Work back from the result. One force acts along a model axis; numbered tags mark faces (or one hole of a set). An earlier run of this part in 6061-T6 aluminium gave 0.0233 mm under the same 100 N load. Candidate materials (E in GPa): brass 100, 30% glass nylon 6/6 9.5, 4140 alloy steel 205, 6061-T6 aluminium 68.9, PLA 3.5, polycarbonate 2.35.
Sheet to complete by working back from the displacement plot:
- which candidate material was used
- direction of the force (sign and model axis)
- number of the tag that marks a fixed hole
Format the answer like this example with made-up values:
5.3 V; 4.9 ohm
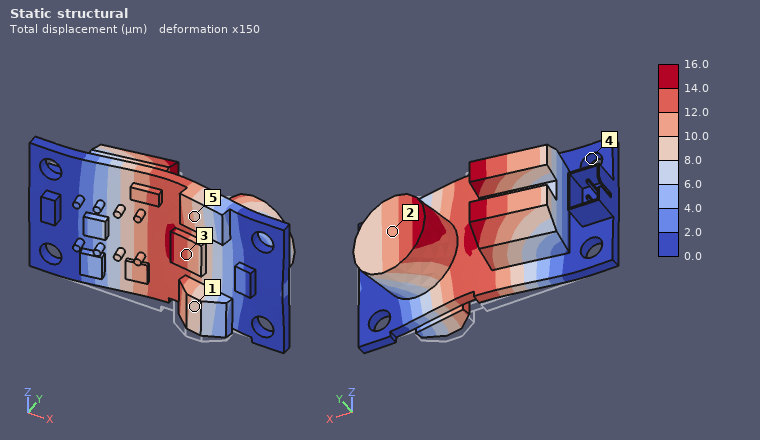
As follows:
brass; +Y; 4
